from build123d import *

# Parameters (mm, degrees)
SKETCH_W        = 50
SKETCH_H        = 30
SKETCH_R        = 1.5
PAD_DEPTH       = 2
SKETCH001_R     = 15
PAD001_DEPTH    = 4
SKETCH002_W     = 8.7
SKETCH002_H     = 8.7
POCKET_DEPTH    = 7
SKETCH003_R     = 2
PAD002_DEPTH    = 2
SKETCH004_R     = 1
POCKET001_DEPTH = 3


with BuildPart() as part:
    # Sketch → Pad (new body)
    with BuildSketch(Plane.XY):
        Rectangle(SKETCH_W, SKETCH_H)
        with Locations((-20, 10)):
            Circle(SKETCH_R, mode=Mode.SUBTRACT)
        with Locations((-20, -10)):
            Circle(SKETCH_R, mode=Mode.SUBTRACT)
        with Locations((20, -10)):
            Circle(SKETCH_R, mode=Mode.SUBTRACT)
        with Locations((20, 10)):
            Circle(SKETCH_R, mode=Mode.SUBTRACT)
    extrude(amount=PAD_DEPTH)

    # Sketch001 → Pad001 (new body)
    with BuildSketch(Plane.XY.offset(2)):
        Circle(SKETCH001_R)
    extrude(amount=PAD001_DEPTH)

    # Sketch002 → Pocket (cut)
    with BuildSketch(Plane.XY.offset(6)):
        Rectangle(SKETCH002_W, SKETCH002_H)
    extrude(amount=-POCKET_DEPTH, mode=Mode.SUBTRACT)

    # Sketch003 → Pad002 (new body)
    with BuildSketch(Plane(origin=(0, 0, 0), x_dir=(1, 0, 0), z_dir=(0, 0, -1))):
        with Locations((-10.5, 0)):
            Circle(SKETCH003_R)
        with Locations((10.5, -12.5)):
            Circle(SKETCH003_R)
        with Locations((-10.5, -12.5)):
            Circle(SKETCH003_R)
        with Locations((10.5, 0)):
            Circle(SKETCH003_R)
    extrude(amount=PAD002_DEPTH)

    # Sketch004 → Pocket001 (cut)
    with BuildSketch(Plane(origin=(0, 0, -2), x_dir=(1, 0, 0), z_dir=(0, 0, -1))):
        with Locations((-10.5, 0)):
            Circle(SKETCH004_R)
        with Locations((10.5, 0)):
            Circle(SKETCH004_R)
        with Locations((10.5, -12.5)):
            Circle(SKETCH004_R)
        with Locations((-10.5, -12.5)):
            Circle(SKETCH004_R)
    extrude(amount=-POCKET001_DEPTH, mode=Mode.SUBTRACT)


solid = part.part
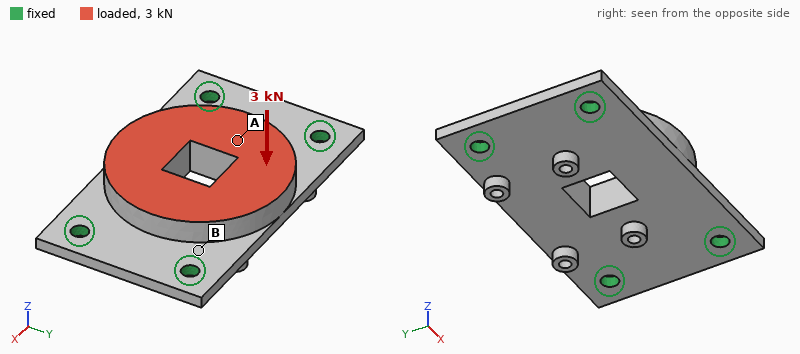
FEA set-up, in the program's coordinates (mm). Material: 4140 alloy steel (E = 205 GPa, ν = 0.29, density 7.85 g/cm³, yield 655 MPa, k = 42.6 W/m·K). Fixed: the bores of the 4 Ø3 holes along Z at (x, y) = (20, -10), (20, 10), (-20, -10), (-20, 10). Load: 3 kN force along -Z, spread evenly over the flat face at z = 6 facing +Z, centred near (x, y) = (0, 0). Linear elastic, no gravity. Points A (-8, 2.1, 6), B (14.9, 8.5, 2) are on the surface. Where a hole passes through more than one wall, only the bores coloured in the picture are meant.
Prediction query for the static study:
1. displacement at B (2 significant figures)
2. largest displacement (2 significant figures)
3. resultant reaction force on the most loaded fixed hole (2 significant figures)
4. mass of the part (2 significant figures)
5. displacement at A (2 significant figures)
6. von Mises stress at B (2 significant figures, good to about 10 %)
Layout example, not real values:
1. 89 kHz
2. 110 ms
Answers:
1. 16 µm
2. 38 µm
3. 1.1 kN
4. 42 g
5. 32 µm
6. 110 MPa
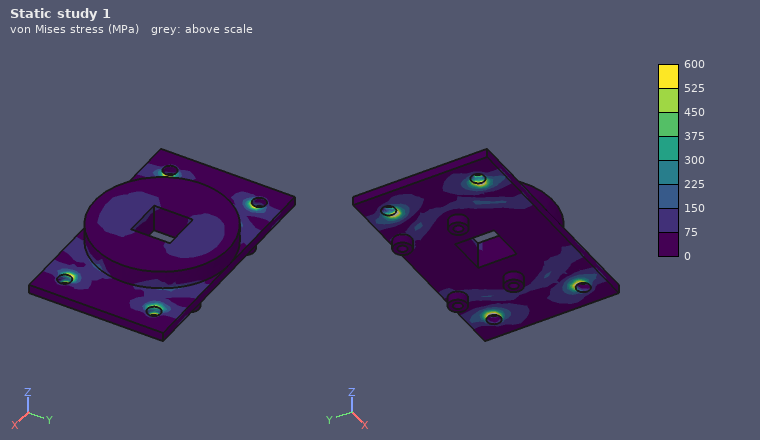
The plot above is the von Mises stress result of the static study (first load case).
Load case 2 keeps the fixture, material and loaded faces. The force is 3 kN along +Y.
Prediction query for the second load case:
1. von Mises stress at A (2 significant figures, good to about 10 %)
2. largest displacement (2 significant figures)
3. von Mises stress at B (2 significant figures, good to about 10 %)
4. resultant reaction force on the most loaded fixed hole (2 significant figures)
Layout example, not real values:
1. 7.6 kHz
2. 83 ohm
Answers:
1. 30 MPa
2. 28 µm
3. 120 MPa
4. 1.0 kN
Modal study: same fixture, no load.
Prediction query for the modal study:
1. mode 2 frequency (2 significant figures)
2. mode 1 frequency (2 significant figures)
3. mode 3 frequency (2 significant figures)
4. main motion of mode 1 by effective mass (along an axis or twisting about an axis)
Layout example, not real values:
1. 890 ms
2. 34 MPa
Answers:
1. 9700 Hz
2. 8400 Hz
3. 18 kHz
4. along Z
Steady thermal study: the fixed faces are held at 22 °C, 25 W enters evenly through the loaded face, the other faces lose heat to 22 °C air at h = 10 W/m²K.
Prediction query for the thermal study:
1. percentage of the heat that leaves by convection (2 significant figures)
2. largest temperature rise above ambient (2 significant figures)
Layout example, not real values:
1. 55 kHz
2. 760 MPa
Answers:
1. 4.4 %
2. 59 K
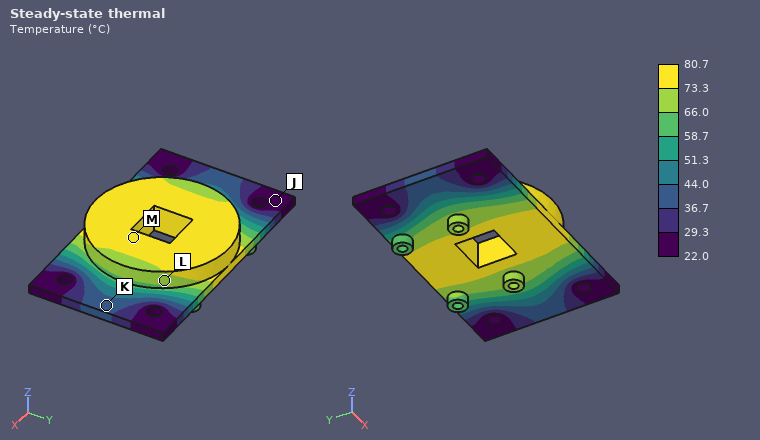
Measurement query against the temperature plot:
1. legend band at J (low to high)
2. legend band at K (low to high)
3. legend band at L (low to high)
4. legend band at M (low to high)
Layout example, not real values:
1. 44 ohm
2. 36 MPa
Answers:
1. 22.0 to 29.3 °C
2. 36.7 to 44.0 °C
3. 66.0 to 73.3 °C
4. 73.3 to 80.7 °C
